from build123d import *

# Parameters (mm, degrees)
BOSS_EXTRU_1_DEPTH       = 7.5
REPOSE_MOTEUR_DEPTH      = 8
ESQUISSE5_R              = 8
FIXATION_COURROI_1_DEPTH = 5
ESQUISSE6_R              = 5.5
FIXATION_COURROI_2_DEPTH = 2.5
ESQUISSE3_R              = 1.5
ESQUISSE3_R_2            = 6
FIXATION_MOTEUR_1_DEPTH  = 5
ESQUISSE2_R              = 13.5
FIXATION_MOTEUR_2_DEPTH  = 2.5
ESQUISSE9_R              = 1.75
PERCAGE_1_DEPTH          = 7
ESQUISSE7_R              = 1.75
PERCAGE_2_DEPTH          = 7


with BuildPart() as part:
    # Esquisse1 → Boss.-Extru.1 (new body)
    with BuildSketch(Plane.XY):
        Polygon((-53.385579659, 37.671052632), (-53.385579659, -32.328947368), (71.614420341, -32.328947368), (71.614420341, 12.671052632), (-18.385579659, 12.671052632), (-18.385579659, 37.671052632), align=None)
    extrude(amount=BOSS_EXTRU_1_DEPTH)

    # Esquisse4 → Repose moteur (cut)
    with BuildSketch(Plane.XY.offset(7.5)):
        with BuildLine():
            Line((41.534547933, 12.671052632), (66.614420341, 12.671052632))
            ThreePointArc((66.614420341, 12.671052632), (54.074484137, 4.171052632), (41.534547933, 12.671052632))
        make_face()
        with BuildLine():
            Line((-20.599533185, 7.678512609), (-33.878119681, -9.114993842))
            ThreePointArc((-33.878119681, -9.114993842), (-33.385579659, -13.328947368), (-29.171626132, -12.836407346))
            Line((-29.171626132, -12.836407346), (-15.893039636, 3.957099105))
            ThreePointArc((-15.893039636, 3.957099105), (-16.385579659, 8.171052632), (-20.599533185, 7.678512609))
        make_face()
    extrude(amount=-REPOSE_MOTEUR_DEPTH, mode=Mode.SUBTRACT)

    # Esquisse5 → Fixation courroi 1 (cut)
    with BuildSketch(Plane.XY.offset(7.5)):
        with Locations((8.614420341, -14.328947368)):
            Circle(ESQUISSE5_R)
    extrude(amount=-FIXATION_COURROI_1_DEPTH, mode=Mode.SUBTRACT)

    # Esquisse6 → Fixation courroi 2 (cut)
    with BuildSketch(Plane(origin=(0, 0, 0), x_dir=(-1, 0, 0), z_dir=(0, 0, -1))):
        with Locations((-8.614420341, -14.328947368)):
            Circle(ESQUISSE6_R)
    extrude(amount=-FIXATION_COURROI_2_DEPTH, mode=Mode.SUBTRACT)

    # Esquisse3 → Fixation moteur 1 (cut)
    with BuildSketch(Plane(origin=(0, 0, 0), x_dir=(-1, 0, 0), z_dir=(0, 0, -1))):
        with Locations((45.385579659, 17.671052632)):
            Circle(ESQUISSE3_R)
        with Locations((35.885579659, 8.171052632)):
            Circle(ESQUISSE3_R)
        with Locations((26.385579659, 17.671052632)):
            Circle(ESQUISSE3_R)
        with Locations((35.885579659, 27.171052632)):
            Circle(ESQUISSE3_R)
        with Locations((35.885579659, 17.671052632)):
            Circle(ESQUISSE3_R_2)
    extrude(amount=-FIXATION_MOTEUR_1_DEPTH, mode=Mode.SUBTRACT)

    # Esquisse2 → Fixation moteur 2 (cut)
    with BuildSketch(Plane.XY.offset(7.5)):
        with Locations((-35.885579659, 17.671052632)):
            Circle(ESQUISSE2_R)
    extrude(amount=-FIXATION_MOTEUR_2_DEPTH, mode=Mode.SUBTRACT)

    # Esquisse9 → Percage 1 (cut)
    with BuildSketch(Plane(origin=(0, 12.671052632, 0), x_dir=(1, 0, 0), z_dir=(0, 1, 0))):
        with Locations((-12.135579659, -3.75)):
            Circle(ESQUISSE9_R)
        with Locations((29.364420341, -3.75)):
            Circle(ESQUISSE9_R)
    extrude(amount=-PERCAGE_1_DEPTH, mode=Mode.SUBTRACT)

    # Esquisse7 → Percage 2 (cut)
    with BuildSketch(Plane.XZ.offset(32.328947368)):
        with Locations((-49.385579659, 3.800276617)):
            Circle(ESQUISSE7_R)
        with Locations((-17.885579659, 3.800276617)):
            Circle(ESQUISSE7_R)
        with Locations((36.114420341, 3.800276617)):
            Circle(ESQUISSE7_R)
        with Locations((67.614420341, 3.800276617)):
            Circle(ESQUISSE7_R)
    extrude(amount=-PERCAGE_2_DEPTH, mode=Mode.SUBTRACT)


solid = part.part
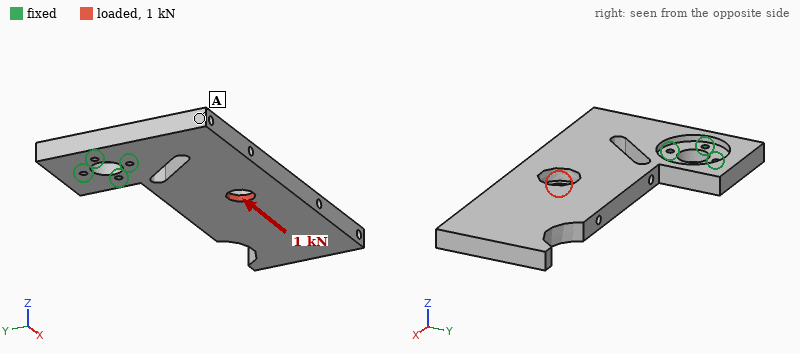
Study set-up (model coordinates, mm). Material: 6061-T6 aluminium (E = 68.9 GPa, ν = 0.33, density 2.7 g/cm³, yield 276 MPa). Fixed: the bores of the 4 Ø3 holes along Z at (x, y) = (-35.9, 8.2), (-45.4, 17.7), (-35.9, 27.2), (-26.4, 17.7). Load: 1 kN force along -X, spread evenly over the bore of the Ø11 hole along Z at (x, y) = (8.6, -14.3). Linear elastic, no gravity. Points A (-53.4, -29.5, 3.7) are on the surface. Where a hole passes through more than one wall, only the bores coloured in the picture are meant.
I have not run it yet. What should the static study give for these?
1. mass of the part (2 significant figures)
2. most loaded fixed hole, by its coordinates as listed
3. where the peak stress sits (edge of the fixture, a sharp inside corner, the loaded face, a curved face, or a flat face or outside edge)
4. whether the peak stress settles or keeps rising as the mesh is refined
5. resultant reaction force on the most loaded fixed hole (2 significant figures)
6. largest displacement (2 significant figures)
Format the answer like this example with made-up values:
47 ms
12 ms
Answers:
120 g
(-35.9, 8.2)
edge of the fixture
keeps rising
1.1 kN
0.19 mm
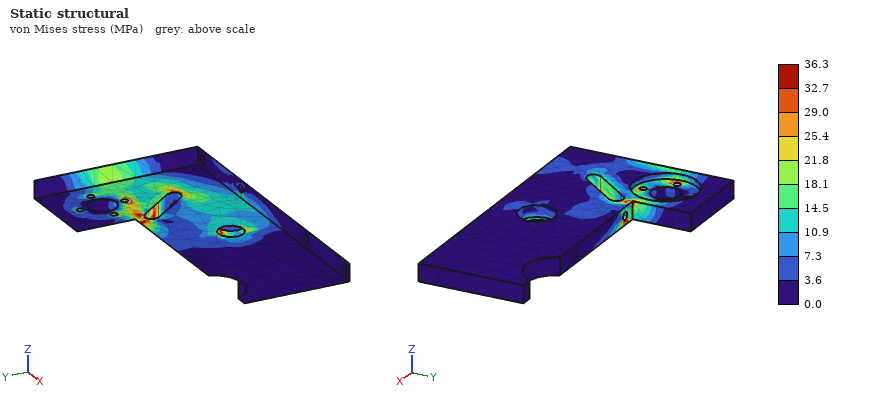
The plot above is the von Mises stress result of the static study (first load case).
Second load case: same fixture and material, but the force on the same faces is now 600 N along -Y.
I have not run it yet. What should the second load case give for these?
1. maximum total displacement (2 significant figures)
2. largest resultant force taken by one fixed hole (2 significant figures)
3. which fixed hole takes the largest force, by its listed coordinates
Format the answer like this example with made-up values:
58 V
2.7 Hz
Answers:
81 µm
1.1 kN
(-26.4, 17.7)
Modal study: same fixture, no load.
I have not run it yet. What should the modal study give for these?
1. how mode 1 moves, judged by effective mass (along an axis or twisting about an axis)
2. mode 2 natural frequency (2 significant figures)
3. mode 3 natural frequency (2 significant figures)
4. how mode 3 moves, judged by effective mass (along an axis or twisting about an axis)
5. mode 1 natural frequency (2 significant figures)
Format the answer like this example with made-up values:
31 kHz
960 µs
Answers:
along Z
1500 Hz
1600 Hz
along Y
370 Hz
